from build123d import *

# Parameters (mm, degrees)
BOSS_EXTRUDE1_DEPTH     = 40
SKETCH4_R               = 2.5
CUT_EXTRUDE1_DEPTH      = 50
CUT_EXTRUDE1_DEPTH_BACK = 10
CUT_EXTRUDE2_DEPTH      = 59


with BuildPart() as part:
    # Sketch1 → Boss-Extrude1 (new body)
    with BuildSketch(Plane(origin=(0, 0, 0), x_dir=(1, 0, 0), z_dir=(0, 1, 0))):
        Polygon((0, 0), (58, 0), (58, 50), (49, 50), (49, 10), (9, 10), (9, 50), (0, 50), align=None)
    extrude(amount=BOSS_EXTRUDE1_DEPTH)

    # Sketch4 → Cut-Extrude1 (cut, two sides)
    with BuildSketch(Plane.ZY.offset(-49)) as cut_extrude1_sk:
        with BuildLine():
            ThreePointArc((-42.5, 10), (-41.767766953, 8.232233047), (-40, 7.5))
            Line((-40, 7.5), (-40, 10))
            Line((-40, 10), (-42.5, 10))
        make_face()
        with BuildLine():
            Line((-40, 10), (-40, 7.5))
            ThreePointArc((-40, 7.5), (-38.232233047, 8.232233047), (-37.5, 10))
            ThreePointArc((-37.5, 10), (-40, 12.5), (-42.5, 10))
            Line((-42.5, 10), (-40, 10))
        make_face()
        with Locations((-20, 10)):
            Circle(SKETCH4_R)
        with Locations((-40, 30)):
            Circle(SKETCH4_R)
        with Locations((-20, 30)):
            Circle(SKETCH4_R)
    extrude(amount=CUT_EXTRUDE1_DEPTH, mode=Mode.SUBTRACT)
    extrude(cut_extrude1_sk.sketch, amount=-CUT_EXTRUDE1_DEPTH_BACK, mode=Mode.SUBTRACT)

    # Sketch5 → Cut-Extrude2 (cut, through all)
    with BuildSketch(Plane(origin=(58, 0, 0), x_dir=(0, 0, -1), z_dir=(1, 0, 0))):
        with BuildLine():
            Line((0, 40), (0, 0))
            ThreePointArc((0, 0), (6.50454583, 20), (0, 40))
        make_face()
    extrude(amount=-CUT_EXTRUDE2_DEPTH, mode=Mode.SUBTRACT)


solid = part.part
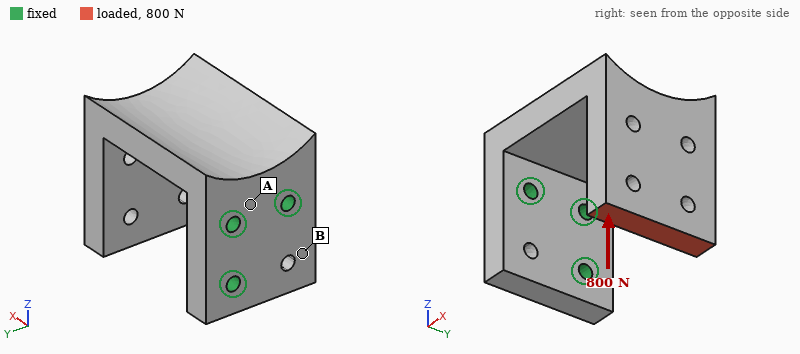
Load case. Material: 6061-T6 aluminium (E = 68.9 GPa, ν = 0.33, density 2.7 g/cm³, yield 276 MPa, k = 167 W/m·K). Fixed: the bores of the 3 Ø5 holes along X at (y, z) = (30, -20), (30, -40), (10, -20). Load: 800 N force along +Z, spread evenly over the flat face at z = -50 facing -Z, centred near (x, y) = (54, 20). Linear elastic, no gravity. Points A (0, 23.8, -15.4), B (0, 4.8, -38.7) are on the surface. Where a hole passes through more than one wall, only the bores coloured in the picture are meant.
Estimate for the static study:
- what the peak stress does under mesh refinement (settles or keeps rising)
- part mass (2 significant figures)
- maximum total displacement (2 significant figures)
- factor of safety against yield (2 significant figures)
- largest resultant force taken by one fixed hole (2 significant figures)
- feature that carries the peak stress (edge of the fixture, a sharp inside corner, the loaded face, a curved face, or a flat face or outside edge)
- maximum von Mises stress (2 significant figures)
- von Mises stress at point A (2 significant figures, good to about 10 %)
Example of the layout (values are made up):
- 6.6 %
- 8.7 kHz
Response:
- settles
- 110 g
- 0.98 mm
- 1.4
- 490 N
- a curved face
- 190 MPa
- 43 MPa
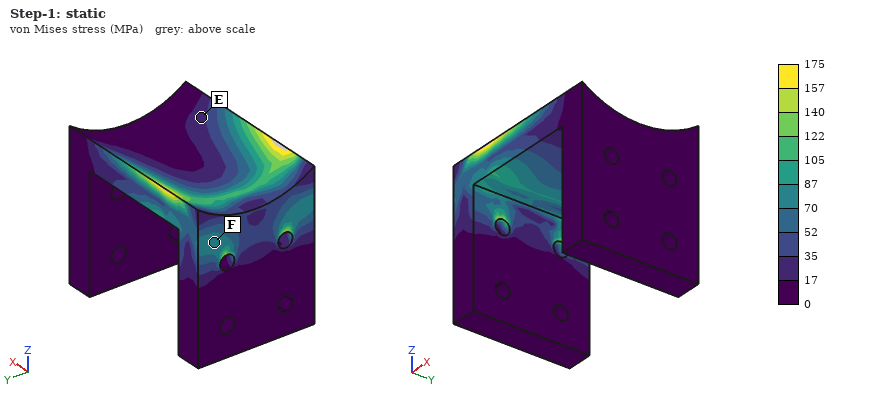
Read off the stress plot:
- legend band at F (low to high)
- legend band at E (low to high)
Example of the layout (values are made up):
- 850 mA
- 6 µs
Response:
- 70 to 87 MPa
- 17 to 35 MPa
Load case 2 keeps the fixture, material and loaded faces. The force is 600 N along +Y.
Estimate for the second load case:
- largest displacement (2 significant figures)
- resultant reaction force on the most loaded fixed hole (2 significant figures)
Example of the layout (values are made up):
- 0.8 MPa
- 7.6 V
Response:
- 0.73 mm
- 1.3 kN
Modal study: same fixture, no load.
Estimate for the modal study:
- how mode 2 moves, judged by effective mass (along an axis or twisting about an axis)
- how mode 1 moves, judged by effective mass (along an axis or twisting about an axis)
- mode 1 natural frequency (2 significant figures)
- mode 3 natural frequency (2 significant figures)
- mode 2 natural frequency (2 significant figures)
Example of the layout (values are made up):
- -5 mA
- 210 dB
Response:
- along Y
- along Z
- 710 Hz
- 2200 Hz
- 1100 Hz
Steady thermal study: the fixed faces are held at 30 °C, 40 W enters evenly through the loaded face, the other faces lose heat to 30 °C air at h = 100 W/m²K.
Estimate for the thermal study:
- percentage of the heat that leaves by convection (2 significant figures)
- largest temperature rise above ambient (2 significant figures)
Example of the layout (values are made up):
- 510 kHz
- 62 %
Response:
- 60 %
- 49 K
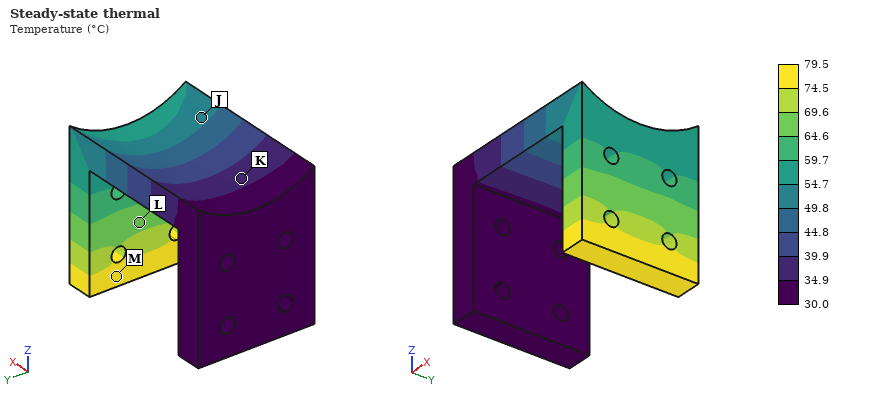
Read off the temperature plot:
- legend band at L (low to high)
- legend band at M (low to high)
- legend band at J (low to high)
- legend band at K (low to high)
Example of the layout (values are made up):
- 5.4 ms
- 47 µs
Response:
- 64.6 to 69.6 °C
- 74.5 to 79.5 °C
- 49.8 to 54.7 °C
- 34.9 to 39.9 °C
